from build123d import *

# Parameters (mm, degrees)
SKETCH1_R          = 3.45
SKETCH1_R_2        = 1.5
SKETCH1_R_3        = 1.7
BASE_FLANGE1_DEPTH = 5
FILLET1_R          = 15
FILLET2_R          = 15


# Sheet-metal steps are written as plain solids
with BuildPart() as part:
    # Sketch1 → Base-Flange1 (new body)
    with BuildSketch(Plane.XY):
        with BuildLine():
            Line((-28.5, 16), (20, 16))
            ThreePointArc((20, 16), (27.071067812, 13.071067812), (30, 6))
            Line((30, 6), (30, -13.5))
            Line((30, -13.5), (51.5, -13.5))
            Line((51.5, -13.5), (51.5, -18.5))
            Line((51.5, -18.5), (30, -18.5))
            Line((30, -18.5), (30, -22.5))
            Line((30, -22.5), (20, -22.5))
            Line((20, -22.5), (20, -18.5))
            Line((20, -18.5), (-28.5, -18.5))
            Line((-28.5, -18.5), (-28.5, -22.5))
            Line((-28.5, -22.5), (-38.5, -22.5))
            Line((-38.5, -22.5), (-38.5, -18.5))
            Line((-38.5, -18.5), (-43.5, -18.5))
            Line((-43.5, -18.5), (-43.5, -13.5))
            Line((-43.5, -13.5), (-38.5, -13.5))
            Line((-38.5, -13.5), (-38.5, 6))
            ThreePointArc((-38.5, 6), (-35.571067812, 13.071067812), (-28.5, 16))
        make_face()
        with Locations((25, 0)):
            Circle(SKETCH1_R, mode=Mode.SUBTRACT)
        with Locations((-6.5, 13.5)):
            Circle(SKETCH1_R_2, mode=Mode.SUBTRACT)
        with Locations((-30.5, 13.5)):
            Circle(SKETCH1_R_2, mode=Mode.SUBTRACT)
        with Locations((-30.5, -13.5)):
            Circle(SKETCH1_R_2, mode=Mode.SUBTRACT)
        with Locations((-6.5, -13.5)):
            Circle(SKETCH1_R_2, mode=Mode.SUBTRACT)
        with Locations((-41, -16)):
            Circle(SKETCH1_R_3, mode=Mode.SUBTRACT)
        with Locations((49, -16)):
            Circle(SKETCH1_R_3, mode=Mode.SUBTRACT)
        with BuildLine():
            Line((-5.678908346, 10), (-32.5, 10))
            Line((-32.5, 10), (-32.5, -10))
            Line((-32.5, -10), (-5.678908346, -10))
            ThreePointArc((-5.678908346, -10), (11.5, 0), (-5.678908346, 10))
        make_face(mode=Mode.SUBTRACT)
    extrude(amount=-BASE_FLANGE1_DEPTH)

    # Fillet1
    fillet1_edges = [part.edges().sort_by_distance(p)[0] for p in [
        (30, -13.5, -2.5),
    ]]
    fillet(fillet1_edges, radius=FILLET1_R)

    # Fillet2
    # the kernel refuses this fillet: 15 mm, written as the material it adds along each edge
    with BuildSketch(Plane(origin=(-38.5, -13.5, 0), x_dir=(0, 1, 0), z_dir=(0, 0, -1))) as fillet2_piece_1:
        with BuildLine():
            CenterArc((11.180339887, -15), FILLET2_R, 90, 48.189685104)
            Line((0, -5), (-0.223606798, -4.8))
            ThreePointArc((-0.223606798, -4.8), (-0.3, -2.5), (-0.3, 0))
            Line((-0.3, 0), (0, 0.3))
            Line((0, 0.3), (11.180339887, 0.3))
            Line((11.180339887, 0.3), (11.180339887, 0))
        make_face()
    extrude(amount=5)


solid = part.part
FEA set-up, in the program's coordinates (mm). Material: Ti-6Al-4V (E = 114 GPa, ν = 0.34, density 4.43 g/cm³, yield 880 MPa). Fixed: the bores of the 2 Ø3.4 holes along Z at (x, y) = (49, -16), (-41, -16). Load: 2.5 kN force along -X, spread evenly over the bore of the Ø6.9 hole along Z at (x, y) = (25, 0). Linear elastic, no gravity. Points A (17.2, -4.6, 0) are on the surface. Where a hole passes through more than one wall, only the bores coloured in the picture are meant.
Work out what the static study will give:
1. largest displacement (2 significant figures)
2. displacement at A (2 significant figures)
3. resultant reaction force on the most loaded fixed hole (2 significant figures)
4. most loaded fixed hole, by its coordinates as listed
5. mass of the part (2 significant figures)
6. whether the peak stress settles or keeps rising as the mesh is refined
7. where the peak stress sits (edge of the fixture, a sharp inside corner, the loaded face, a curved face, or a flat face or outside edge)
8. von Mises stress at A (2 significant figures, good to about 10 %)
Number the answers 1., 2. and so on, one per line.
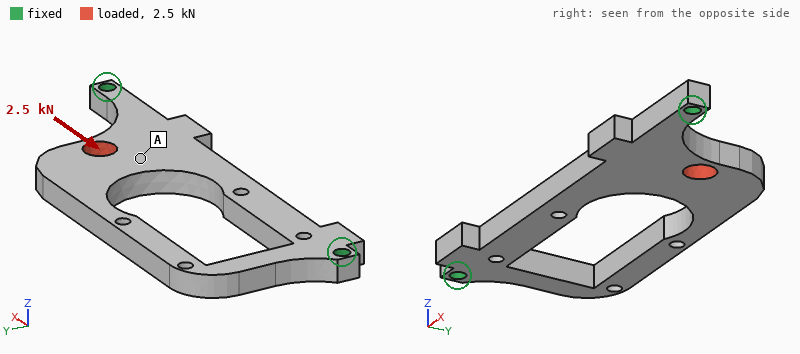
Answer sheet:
1. 93 µm
2. 55 µm
3. 1.4 kN
4. (49, -16)
5. 36 g
6. keeps rising
7. a sharp inside corner
8. 38 MPa
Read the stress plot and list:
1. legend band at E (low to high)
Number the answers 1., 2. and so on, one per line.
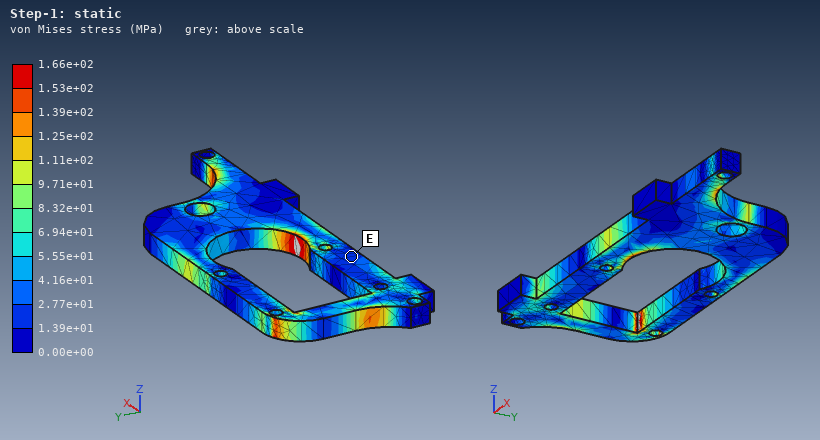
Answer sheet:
1. 1.39e+01 to 2.77e+01 MPa
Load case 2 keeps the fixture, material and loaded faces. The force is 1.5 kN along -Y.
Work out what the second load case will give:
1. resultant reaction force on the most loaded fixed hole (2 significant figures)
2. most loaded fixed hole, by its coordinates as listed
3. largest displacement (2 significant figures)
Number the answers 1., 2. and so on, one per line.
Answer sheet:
1. 1.3 kN
2. (49, -16)
3. 85 µm
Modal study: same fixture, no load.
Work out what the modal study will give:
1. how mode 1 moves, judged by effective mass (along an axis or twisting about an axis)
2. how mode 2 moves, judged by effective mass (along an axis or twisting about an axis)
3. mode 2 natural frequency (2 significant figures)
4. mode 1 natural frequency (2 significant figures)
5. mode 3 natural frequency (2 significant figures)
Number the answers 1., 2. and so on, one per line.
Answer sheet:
1. along Z
2. along Z
3. 3300 Hz
4. 1400 Hz
5. 4000 Hz
